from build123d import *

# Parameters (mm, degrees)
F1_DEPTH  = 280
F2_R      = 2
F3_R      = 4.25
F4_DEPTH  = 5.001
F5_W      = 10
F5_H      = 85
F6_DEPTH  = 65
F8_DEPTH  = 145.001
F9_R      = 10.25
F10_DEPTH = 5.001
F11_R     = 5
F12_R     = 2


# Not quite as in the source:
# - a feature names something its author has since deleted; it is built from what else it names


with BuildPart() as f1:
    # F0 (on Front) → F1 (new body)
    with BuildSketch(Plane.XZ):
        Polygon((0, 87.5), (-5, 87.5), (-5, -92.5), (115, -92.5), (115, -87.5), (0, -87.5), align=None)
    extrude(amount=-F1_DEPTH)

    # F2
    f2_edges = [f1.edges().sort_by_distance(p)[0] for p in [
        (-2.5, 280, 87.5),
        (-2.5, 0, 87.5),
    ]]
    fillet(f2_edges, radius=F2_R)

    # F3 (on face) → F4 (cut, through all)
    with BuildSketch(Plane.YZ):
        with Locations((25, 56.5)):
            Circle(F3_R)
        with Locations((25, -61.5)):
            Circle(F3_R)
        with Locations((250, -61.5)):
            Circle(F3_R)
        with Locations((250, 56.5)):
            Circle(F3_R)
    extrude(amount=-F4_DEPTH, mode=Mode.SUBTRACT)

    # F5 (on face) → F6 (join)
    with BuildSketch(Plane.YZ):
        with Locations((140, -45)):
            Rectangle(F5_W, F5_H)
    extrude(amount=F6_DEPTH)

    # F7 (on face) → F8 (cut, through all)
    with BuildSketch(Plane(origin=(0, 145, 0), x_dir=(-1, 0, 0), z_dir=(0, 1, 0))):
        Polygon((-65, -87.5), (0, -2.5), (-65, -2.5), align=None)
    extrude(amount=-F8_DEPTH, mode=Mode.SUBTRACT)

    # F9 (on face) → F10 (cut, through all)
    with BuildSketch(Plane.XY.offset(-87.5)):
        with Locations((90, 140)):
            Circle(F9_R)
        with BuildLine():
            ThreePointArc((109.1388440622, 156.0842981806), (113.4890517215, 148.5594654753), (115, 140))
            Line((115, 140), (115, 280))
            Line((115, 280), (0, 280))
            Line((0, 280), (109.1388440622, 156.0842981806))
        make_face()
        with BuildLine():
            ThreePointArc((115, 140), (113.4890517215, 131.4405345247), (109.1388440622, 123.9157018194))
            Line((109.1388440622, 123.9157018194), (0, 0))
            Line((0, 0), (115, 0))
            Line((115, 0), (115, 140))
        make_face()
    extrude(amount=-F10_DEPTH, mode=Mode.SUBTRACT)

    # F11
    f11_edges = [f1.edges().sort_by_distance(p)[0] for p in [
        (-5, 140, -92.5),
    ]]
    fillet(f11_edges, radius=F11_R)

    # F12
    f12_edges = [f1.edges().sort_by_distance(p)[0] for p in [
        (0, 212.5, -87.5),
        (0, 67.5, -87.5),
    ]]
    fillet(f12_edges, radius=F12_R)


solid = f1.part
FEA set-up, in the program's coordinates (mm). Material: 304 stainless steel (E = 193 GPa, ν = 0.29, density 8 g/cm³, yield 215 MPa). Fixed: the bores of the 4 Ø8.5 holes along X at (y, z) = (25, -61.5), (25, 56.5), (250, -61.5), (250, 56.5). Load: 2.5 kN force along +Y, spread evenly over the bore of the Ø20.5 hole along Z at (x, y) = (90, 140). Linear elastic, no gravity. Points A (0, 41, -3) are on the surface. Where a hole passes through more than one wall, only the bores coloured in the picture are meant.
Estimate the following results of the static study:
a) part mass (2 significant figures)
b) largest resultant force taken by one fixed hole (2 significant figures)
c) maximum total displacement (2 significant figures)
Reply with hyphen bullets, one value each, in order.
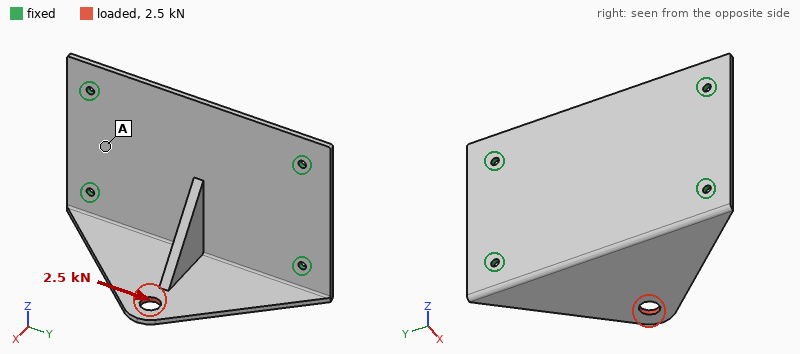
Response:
- 2.9 kg
- 1.6 kN
- 77 µm
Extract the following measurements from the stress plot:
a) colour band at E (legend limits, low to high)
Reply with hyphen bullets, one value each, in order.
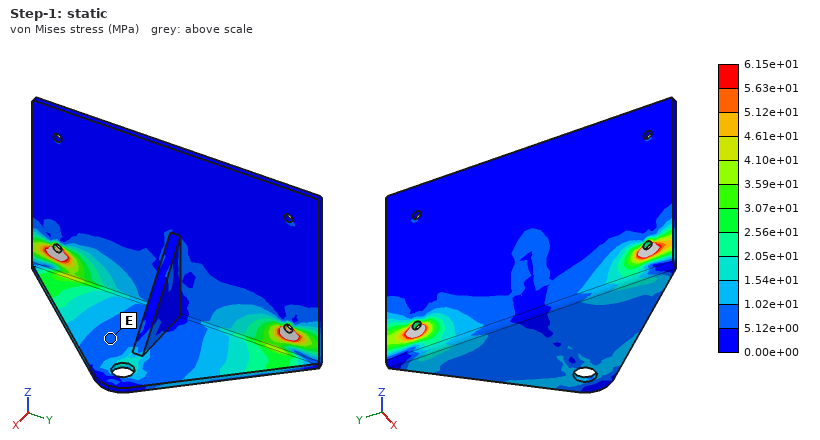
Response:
- 5.12e+00 to 1.02e+01 MPa
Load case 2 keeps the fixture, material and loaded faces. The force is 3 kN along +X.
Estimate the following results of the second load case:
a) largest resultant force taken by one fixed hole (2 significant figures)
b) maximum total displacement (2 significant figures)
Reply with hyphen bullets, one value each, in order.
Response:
- 2.1 kN
- 0.18 mm
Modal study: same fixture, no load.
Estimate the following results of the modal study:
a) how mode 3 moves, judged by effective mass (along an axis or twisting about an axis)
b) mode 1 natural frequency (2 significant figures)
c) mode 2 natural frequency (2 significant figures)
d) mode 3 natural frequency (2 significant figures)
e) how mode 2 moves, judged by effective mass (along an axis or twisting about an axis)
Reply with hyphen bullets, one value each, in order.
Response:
- along X
- 430 Hz
- 760 Hz
- 910 Hz
- along X
